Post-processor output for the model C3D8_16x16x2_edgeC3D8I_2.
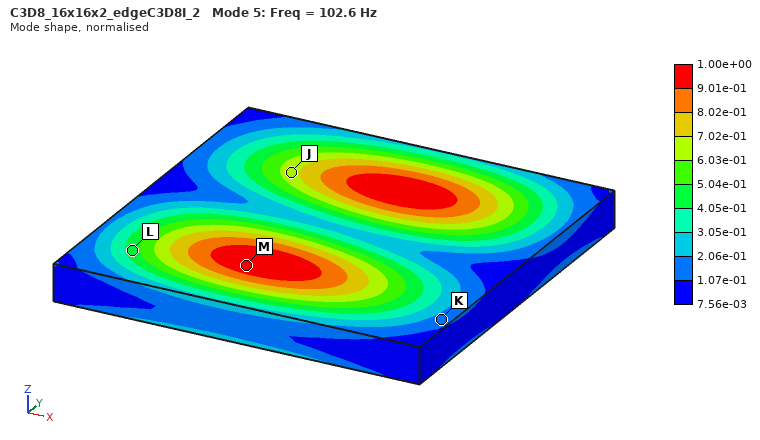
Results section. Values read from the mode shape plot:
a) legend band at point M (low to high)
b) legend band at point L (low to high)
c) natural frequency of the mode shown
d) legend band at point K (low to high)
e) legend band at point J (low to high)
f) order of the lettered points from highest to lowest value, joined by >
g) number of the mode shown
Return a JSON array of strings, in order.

["9.01e-01 to 1.00e+00", "4.05e-01 to 5.04e-01", "102.6 Hz", "1.07e-01 to 2.06e-01", "6.03e-01 to 7.02e-01", "M > J > L > K", "5"]
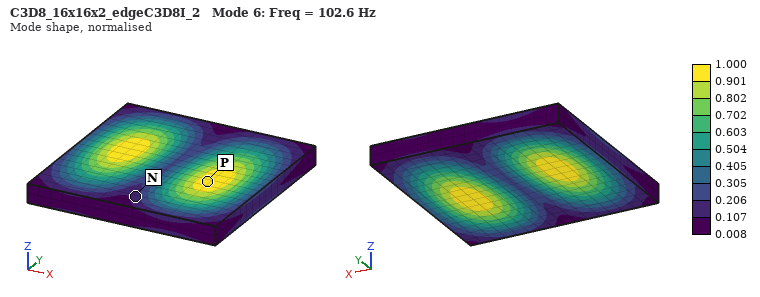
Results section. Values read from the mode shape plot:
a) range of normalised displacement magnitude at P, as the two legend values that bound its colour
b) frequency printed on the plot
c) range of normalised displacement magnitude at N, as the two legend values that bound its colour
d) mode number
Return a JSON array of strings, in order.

["0.901 to 1.000", "102.6 Hz", "0.107 to 0.206", "6"]
